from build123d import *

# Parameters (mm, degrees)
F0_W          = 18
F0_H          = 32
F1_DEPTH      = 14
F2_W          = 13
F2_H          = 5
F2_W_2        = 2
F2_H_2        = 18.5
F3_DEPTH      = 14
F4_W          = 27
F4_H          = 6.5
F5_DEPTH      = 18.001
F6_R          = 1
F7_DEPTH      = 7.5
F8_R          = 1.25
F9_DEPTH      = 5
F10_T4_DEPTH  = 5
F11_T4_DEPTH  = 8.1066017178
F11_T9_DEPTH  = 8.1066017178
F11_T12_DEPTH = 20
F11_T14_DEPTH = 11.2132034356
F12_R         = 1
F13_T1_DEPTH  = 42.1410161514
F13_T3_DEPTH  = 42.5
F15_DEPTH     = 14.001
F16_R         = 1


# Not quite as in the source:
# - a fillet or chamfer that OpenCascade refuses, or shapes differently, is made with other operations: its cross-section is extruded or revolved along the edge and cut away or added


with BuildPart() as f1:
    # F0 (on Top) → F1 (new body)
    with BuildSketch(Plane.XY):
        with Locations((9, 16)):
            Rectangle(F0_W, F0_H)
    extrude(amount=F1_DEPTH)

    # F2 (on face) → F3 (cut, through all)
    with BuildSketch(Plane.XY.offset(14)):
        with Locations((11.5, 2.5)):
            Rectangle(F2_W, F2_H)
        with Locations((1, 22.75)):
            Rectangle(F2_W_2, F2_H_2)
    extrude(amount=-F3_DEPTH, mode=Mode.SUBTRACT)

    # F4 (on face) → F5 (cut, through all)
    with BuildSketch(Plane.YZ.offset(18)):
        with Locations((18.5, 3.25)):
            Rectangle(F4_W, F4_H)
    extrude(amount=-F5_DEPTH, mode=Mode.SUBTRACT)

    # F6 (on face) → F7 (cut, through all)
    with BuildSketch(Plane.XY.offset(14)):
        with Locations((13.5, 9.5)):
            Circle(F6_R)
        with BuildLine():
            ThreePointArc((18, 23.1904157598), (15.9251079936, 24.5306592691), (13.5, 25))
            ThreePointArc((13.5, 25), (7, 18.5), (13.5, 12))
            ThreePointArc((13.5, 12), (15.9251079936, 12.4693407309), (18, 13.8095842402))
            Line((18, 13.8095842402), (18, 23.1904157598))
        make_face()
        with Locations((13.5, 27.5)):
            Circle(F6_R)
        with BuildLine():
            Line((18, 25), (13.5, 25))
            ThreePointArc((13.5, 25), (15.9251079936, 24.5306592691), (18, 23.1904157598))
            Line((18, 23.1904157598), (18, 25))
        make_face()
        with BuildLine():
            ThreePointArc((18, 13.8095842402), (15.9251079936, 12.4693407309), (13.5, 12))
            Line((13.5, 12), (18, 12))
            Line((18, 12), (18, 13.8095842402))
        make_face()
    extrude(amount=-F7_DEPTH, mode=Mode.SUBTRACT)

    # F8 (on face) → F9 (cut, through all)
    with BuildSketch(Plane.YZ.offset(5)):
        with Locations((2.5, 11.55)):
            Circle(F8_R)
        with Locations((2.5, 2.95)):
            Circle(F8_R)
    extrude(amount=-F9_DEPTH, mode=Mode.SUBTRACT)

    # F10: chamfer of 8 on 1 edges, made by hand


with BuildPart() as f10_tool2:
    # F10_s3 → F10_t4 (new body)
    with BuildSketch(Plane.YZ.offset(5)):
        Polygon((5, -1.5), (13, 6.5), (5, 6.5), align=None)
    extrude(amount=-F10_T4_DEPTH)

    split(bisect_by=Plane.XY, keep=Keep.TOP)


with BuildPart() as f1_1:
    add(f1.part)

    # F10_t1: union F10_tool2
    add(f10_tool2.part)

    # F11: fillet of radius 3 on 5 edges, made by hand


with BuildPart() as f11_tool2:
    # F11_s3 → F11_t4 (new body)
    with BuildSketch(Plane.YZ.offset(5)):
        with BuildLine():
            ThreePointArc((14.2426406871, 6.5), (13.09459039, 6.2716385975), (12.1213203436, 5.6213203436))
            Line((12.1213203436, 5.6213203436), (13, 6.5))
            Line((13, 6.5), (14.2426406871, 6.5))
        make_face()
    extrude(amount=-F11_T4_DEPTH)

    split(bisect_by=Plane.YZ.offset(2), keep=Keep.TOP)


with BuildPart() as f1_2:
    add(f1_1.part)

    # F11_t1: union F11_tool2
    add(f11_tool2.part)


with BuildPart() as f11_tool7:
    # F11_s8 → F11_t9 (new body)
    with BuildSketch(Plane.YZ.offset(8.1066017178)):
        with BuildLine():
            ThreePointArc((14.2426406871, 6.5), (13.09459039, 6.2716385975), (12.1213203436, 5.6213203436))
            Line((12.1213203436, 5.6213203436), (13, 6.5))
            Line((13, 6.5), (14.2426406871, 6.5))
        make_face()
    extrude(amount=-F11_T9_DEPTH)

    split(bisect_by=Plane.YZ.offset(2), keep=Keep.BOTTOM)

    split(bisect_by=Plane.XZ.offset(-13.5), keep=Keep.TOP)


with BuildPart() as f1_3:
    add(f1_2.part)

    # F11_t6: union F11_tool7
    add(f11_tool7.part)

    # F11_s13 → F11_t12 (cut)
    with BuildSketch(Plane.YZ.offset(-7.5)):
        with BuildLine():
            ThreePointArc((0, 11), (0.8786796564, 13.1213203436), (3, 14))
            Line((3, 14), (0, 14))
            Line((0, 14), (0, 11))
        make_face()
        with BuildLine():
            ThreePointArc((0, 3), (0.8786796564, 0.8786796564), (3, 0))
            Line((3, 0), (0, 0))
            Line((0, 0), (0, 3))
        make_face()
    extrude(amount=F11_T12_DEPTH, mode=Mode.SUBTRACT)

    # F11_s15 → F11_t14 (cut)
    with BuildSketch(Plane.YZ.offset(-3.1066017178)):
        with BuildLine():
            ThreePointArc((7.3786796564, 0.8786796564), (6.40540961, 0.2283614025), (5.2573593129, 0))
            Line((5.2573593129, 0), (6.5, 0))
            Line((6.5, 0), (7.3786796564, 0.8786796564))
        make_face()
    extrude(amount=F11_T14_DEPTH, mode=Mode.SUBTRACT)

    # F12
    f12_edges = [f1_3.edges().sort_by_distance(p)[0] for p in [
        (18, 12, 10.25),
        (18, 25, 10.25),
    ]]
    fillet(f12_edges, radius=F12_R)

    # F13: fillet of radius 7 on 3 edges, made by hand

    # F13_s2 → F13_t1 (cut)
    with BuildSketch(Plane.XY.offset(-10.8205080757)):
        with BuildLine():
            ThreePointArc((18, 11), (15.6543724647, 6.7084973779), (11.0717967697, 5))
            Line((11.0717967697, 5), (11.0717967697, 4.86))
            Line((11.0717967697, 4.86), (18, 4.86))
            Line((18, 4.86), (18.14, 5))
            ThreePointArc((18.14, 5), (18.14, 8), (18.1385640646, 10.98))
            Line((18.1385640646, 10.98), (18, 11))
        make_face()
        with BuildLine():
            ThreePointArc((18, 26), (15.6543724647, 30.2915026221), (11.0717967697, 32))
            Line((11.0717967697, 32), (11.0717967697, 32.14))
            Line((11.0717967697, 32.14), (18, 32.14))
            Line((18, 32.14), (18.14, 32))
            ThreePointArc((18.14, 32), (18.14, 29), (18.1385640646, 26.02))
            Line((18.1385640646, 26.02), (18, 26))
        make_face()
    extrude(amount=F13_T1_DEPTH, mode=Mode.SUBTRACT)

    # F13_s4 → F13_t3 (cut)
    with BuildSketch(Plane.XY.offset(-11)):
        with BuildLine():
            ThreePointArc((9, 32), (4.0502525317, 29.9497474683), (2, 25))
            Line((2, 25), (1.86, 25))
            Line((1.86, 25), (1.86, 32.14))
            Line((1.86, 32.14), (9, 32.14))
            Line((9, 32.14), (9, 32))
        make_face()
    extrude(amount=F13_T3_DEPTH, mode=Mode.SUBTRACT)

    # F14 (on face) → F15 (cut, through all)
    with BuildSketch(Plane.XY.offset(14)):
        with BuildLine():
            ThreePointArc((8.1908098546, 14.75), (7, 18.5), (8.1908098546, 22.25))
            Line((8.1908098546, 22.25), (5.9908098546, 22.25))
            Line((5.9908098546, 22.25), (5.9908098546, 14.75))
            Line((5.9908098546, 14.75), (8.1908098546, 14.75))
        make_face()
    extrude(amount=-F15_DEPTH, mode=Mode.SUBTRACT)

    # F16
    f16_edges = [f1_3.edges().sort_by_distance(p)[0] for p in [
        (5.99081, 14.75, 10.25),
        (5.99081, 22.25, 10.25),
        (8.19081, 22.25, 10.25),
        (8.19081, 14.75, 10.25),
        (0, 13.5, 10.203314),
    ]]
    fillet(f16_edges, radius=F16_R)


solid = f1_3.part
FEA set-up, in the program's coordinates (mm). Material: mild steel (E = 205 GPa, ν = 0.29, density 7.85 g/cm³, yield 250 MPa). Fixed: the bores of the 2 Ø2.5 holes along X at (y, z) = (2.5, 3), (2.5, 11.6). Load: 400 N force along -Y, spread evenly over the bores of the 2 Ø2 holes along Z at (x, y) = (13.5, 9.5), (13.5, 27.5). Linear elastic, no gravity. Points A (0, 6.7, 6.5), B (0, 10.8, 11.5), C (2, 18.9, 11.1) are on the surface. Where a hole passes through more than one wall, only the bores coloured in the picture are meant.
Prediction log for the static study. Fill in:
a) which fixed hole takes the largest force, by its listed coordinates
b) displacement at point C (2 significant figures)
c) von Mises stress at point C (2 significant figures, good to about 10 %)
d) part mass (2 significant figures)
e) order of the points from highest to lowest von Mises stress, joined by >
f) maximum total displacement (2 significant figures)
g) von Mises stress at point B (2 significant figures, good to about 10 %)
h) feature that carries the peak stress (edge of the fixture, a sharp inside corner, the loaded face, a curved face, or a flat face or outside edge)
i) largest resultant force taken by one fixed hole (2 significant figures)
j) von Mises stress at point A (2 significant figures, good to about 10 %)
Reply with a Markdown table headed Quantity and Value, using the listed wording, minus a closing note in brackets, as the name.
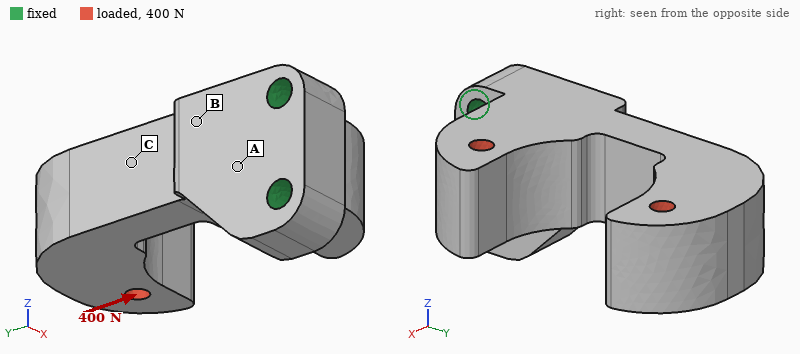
| Quantity | Value |
|---|---|
| which fixed hole takes the largest force, by its listed coordinates | (2.5, 11.6) |
| displacement at point C | 17 µm |
| von Mises stress at point C | 87 MPa |
| part mass | 20 g |
| order of the points from highest to lowest von Mises stress, joined by > | C > A > B |
| maximum total displacement | 67 µm |
| von Mises stress at point B | 19 MPa |
| feature that carries the peak stress | edge of the fixture |
| largest resultant force taken by one fixed hole | 340 N |
| von Mises stress at point A | 51 MPa |
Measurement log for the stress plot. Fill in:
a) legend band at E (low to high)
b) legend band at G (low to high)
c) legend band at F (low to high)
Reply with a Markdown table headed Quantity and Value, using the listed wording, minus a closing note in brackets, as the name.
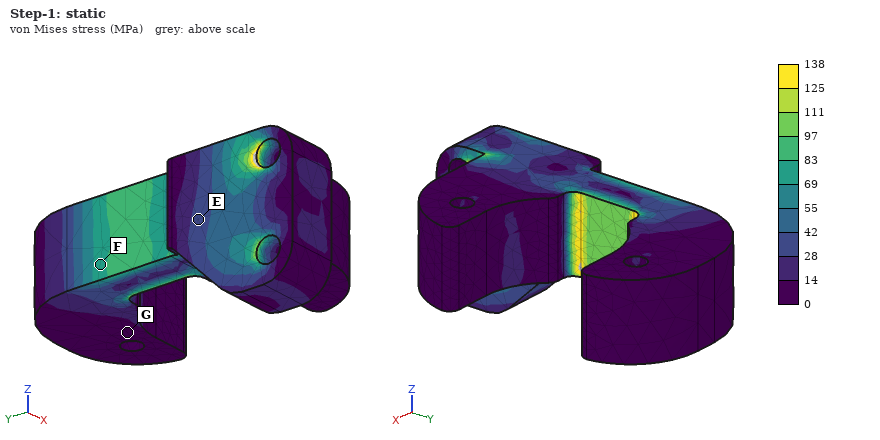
| Quantity | Value |
|---|---|
| legend band at E | 28 to 42 MPa |
| legend band at G | 0 to 14 MPa |
| legend band at F | 69 to 83 MPa |
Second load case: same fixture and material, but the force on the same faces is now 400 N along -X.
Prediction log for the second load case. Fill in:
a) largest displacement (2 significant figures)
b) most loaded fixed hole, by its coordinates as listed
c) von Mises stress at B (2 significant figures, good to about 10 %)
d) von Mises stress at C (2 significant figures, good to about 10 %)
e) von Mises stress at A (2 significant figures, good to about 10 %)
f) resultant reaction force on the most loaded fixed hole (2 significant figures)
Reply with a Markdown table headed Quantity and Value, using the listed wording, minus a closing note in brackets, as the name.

| Quantity | Value |
|---|---|
| largest displacement | 74 µm |
| most loaded fixed hole, by its coordinates as listed | (2.5, 11.6) |
| von Mises stress at B | 26 MPa |
| von Mises stress at C | 85 MPa |
| von Mises stress at A | 66 MPa |
| resultant reaction force on the most loaded fixed hole | 280 N |
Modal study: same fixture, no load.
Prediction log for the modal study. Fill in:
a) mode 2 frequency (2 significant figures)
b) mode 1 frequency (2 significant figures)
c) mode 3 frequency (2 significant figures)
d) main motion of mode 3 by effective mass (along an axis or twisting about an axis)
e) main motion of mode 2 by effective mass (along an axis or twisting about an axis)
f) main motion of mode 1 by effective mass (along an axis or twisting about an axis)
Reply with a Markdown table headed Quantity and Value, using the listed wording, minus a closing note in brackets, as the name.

| Quantity | Value |
|---|---|
| mode 2 frequency | 5600 Hz |
| mode 1 frequency | 3600 Hz |
| mode 3 frequency | 13 kHz |
| main motion of mode 3 by effective mass | along X |
| main motion of mode 2 by effective mass | along Z |
| main motion of mode 1 by effective mass | along X |
